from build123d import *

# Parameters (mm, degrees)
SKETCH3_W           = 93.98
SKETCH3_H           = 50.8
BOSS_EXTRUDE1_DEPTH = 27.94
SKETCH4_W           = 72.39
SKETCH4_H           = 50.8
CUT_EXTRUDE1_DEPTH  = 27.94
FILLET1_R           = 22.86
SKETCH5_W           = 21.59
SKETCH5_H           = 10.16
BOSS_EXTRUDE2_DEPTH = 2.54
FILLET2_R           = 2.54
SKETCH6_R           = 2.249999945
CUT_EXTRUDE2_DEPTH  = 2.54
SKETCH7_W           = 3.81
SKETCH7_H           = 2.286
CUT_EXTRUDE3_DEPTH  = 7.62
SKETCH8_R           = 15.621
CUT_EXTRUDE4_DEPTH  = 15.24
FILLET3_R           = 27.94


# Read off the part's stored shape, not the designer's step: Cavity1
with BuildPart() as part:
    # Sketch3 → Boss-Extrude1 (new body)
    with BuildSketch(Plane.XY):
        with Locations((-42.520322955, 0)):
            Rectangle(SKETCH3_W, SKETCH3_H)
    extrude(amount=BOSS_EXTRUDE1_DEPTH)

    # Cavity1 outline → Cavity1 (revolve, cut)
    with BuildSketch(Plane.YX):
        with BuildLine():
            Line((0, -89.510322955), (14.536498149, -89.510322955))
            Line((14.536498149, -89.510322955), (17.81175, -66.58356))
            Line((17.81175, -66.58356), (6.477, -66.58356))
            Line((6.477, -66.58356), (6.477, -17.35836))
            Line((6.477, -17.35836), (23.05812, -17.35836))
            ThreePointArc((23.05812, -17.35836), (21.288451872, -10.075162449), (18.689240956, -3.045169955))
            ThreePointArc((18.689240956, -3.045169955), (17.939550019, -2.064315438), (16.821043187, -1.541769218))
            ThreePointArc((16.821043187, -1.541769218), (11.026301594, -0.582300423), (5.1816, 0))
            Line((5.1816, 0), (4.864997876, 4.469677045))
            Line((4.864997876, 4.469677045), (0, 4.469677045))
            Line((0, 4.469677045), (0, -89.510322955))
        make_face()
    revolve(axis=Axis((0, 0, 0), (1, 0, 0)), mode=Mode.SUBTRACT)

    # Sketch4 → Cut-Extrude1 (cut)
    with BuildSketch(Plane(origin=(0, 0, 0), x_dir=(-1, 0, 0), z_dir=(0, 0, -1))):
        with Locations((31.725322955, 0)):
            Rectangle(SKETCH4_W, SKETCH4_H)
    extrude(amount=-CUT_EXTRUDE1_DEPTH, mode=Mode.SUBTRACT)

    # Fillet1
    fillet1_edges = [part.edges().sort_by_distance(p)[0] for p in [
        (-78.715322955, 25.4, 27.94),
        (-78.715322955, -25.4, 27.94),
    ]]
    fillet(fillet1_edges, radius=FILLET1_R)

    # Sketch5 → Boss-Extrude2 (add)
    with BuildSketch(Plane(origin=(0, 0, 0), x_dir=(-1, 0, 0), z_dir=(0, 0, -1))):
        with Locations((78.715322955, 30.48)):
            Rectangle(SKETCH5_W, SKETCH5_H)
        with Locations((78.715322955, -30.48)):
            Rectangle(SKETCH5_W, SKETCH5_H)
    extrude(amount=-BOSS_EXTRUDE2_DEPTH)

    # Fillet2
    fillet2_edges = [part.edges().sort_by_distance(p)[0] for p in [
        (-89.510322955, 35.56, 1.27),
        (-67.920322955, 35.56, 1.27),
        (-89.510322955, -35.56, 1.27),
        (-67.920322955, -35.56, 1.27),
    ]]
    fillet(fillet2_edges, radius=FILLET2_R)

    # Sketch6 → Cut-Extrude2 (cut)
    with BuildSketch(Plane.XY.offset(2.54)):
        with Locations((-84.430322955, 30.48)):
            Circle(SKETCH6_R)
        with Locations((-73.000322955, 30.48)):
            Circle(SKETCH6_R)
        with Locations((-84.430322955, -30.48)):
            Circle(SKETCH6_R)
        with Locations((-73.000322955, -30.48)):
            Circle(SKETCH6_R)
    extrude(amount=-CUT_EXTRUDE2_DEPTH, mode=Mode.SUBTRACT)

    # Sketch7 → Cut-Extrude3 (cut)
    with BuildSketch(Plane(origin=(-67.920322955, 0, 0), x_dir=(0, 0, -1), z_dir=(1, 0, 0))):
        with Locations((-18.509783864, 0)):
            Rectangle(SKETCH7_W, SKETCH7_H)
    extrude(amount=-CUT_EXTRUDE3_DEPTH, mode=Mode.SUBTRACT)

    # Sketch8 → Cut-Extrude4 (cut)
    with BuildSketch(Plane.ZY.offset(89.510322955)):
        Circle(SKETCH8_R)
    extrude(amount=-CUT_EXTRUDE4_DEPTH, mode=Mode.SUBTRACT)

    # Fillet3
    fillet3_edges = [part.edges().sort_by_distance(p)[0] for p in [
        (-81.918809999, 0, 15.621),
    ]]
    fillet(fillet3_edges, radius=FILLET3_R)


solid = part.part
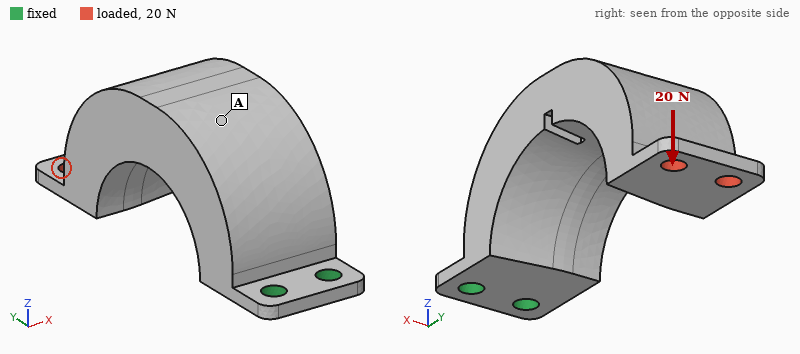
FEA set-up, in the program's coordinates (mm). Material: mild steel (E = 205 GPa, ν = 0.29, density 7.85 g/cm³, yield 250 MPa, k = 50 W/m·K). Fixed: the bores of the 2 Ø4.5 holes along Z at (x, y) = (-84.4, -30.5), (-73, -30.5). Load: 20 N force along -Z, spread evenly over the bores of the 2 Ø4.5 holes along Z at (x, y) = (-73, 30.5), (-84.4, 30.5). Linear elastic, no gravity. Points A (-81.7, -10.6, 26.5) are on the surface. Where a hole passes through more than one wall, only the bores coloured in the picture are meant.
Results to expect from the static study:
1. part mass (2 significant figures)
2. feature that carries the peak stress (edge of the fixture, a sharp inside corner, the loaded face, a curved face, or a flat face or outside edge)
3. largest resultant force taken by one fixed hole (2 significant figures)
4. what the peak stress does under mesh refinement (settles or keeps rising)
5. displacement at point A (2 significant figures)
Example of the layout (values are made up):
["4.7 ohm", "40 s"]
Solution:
["140 g", "edge of the fixture", "10 N", "keeps rising", "28 µm"]
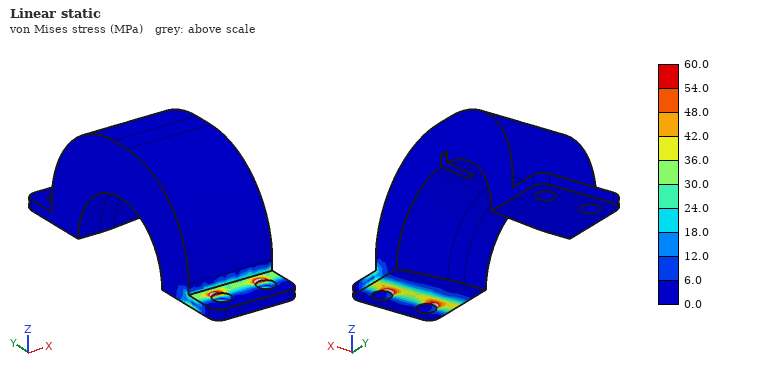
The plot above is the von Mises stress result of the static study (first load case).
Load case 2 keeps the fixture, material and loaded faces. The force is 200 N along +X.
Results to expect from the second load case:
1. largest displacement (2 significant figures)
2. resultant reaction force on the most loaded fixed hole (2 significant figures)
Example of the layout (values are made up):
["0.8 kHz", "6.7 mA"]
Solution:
["46 µm", "860 N"]
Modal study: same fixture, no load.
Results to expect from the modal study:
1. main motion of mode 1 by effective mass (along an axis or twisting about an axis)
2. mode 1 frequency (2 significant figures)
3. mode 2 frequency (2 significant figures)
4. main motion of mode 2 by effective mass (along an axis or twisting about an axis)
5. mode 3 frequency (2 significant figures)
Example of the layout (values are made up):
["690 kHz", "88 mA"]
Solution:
["along Z", "430 Hz", "1900 Hz", "along X", "3300 Hz"]
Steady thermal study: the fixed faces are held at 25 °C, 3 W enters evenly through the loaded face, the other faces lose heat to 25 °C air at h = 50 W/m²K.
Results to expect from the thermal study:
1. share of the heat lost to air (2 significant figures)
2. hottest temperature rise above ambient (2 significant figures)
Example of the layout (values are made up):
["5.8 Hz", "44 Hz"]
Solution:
["64 %", "21 K"]
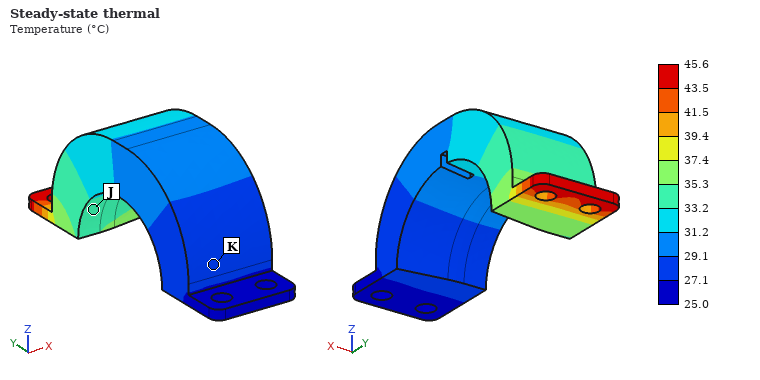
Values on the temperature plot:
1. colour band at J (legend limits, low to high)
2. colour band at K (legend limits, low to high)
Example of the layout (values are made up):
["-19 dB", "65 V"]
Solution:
["33.2 to 35.3 °C", "27.1 to 29.1 °C"]
